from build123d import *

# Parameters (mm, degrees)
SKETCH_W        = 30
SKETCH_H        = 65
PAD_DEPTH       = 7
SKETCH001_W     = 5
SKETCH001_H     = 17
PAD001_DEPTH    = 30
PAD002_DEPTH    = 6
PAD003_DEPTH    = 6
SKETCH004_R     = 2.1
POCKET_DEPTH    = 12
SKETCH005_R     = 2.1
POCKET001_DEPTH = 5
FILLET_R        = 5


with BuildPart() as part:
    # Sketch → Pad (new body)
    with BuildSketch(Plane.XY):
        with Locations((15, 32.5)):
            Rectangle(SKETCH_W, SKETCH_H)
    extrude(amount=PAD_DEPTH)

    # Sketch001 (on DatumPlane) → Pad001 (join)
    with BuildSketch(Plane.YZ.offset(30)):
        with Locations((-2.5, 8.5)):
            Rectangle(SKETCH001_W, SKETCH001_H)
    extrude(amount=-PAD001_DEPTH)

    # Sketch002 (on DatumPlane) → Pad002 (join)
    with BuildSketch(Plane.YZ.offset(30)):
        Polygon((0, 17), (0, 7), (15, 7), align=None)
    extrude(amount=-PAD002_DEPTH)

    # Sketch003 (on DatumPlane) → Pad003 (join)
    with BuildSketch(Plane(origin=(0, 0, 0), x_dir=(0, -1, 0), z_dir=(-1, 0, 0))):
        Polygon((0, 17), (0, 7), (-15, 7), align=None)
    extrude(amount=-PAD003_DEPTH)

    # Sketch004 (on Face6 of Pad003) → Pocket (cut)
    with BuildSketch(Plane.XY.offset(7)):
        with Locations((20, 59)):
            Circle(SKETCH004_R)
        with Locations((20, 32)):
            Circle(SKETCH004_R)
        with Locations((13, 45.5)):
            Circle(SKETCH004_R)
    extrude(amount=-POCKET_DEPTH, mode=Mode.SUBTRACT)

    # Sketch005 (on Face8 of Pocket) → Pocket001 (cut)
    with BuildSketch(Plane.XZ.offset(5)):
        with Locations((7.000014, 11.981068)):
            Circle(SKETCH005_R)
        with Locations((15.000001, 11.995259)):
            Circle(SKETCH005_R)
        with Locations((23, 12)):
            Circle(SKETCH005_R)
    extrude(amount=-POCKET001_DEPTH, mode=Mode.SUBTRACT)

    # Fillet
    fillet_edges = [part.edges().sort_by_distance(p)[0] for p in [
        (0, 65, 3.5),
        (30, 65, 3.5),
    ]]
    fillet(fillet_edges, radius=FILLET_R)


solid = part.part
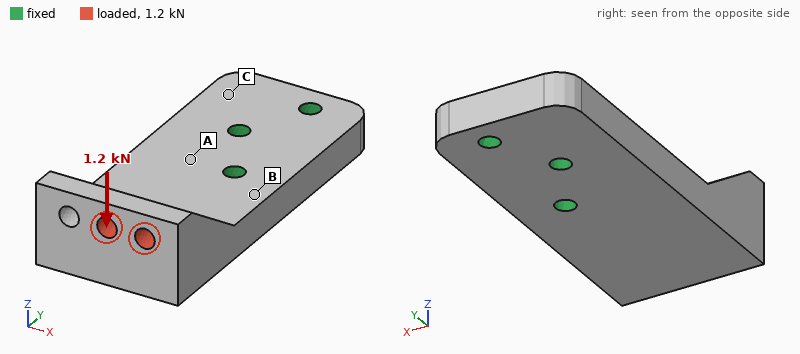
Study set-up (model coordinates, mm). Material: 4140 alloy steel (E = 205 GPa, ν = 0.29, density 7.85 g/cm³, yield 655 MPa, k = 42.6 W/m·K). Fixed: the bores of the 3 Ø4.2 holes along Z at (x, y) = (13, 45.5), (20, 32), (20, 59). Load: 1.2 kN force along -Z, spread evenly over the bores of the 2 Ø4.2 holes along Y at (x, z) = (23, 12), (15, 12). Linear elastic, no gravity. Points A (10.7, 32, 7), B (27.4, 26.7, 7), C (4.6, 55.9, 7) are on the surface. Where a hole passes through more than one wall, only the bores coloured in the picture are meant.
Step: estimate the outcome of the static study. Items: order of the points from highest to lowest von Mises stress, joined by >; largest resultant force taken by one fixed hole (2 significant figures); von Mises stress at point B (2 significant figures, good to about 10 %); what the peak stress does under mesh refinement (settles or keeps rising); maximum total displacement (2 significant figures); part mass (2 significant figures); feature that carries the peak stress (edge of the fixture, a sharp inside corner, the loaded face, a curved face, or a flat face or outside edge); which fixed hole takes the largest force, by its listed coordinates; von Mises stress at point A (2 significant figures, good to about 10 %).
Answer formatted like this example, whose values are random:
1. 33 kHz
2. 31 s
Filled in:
1. B > A > C
2. 2.2 kN
3. 140 MPa
4. keeps rising
5. 0.13 mm
6. 130 g
7. edge of the fixture
8. (20, 32)
9. 92 MPa
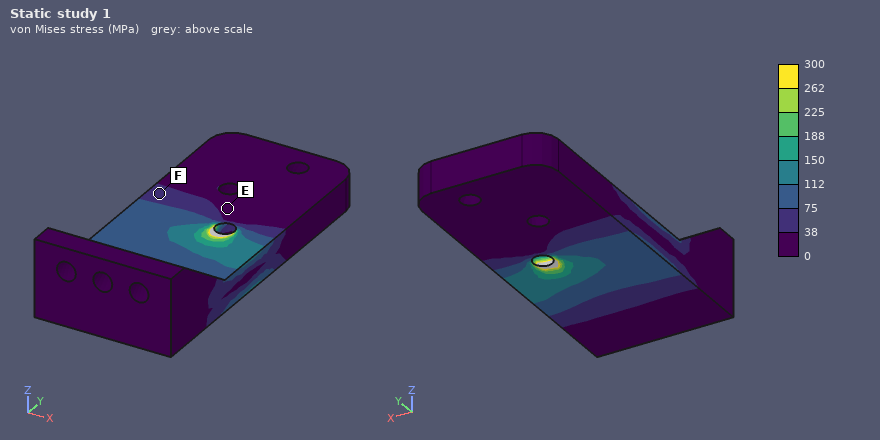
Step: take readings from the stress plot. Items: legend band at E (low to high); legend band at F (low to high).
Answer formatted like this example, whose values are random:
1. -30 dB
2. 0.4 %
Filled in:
1. 0 to 38 MPa
2. 38 to 75 MPa
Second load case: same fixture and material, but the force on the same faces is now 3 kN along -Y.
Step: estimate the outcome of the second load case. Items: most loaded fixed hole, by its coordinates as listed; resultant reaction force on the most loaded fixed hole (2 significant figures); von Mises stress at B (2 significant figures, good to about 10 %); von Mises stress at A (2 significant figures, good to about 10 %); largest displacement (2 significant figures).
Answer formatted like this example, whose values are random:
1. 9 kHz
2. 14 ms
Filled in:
1. (20, 32)
2. 2.3 kN
3. 120 MPa
4. 72 MPa
5. 0.12 mm
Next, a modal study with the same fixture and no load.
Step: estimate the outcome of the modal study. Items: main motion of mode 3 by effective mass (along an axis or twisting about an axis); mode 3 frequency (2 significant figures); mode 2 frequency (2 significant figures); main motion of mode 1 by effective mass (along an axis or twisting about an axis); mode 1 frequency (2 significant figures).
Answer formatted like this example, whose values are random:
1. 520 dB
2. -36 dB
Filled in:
1. along X
2. 8000 Hz
3. 6000 Hz
4. along Z
5. 2800 Hz
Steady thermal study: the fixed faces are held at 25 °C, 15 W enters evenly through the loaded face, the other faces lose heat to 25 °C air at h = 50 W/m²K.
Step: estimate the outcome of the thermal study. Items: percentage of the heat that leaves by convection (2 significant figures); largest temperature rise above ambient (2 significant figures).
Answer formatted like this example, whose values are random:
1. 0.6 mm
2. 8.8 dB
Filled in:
1. 38 %
2. 61 K
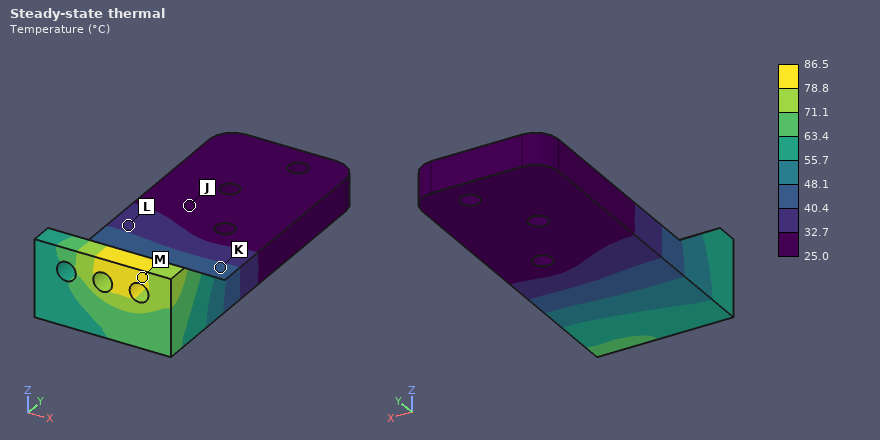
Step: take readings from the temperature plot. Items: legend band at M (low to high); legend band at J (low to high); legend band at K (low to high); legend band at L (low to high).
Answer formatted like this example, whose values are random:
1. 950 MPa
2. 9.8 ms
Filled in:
1. 78.8 to 86.5 °C
2. 25.0 to 32.7 °C
3. 40.4 to 48.1 °C
4. 32.7 to 40.4 °C
